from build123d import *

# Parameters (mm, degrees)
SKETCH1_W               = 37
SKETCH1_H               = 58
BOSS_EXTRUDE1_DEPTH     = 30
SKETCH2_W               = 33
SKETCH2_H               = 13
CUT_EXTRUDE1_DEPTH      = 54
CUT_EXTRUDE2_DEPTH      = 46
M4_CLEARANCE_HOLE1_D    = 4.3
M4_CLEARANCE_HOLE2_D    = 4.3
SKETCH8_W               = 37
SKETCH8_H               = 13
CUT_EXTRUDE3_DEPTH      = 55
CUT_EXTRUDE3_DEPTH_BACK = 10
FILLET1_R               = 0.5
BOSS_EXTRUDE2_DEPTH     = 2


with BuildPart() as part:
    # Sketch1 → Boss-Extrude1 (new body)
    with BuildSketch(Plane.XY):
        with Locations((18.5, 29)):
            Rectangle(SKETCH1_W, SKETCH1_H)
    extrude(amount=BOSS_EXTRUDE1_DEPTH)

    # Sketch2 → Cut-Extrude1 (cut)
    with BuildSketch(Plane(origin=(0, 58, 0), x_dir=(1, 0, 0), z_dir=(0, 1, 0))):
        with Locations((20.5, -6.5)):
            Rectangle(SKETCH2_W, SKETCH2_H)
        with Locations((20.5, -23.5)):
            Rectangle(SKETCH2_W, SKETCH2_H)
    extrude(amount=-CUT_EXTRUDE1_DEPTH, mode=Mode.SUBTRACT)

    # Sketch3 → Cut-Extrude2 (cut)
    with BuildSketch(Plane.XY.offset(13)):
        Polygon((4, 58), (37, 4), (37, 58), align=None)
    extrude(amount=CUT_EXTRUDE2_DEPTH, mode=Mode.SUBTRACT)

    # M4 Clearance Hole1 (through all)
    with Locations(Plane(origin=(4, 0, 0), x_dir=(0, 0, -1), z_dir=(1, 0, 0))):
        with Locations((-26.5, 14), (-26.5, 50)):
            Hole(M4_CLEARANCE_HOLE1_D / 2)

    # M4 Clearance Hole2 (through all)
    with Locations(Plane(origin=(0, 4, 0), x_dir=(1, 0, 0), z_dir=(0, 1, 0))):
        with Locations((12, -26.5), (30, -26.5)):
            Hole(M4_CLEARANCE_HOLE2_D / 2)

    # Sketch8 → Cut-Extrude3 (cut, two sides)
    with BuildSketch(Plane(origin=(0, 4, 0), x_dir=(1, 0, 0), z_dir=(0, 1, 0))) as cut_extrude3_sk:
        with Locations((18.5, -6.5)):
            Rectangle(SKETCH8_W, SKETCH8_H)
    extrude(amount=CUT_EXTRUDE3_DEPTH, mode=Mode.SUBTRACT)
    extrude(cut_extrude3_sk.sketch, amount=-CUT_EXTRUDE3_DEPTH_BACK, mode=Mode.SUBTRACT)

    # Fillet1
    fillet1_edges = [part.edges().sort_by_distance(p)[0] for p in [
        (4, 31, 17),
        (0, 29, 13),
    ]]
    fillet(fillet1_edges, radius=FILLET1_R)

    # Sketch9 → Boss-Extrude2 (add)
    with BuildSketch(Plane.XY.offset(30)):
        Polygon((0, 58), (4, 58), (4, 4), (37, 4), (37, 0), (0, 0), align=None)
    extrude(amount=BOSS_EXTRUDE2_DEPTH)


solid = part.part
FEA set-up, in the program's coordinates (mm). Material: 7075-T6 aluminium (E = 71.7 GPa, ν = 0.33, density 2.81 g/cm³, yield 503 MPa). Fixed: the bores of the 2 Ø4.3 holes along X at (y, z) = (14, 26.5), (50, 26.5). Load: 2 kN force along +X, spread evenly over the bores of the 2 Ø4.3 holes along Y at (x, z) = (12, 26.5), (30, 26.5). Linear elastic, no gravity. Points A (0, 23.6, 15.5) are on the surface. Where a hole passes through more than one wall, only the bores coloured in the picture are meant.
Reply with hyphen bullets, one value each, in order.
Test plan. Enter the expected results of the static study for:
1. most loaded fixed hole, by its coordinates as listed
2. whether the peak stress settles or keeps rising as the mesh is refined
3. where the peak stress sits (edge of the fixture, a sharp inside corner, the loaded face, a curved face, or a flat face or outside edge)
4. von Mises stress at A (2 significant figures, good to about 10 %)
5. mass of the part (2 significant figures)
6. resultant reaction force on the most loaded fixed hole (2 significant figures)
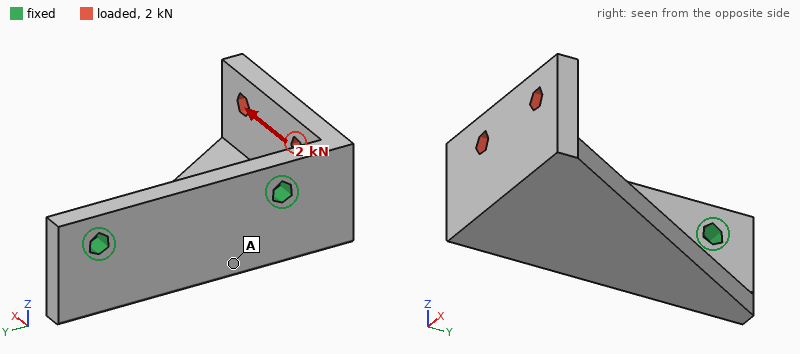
- (14, 26.5)
- keeps rising
- edge of the fixture
- 28 MPa
- 29 g
- 2.4 kN
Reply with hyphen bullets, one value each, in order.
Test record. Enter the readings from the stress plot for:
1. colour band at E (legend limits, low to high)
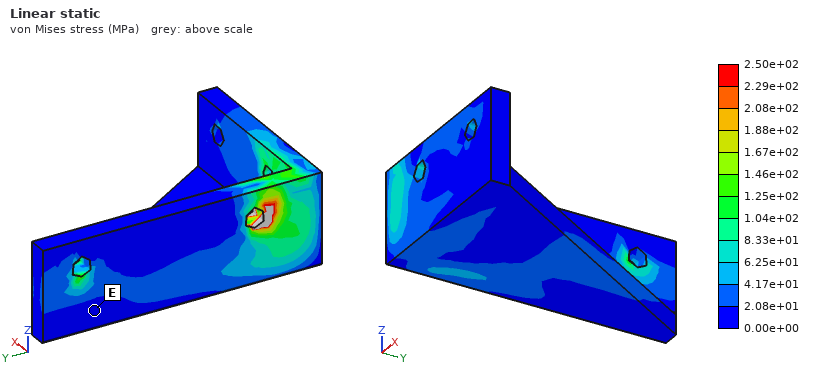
- 0.00e+00 to 2.08e+01 MPa
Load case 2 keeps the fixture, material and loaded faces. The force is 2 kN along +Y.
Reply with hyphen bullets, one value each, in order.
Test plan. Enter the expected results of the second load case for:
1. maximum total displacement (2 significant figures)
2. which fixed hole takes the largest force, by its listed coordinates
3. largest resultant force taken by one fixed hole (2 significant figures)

- 0.53 mm
- (14, 26.5)
- 1.9 kN
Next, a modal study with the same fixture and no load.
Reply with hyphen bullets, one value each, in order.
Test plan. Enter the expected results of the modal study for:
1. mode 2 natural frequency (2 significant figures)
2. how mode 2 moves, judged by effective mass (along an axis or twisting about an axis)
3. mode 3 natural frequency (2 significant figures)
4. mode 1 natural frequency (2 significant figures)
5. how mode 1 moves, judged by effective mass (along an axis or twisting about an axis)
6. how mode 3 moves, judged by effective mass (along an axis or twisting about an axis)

- 5300 Hz
- along Y
- 8300 Hz
- 2600 Hz
- along Z
- along X
